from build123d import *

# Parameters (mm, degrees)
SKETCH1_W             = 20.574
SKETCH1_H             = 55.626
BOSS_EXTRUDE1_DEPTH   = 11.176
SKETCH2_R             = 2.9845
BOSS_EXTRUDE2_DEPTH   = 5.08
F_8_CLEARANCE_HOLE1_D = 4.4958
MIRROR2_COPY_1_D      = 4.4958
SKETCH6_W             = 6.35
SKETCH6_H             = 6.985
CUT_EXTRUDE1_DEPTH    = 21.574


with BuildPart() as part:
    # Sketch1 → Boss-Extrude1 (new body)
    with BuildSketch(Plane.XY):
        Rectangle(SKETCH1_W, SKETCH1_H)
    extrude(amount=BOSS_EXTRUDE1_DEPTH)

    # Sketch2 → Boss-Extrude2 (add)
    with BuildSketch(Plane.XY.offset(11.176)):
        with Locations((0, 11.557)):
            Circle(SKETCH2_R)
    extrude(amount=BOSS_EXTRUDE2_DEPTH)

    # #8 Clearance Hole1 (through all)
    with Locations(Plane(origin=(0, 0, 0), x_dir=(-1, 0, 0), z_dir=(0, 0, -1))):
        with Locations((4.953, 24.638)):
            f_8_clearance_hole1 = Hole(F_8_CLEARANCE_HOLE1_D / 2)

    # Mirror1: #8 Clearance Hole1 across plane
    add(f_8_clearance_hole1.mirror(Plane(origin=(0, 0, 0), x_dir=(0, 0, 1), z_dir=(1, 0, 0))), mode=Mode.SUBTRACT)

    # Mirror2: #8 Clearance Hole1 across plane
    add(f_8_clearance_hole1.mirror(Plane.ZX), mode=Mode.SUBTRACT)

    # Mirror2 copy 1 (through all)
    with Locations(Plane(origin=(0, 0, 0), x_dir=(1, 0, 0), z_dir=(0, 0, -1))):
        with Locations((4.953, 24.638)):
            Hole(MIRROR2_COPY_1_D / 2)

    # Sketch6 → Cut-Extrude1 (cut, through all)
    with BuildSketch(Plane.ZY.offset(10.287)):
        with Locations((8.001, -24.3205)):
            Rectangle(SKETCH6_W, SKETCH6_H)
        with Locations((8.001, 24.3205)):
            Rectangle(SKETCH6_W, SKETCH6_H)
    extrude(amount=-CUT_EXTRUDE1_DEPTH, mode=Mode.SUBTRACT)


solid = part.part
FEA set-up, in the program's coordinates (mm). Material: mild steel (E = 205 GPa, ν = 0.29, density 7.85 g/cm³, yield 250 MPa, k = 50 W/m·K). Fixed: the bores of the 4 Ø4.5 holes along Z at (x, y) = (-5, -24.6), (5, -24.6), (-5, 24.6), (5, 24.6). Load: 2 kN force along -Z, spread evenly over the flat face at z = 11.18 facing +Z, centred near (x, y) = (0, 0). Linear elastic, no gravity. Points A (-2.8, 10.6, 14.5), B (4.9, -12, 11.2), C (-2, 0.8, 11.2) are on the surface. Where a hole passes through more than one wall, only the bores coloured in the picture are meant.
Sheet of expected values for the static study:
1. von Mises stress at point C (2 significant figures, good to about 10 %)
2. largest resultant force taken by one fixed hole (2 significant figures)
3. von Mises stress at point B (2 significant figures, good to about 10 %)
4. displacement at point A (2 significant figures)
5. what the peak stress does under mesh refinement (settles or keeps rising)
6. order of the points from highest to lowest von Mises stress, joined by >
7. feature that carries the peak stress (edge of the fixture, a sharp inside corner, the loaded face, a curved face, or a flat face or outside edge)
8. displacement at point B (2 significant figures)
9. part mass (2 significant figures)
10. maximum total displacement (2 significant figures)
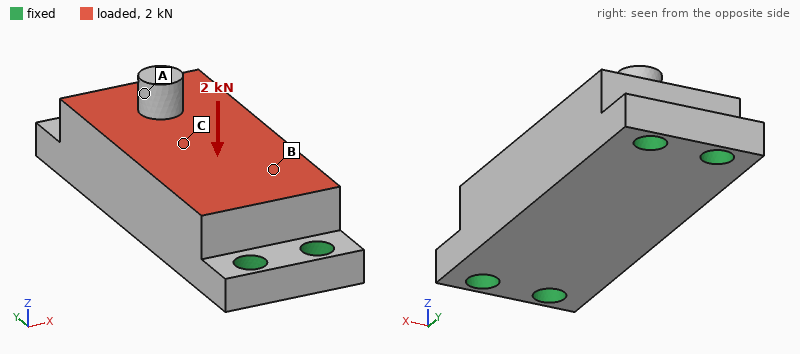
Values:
19 MPa
660 N
11 MPa
3.0 µm
keeps rising
C > B > A
edge of the fixture
2.7 µm
85 g
3.8 µm
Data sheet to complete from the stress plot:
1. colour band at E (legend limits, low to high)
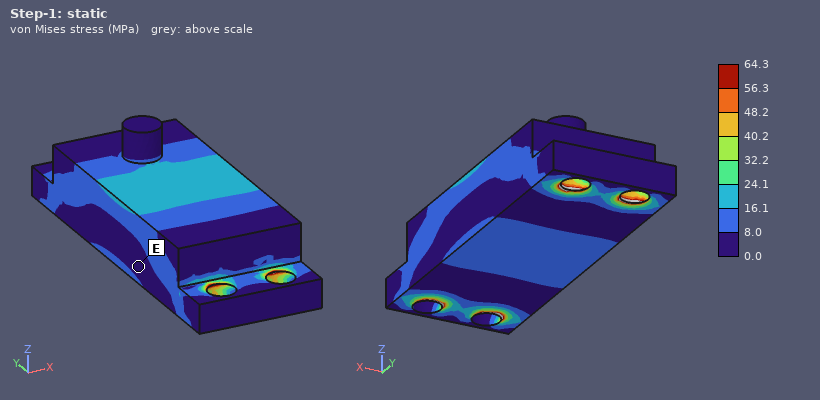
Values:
0.0 to 8.0 MPa
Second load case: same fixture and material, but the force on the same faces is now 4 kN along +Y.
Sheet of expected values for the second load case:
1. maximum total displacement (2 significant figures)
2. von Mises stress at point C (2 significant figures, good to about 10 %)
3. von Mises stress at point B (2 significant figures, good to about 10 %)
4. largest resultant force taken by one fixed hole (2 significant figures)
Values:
1.9 µm
8.4 MPa
8.8 MPa
1.1 kN
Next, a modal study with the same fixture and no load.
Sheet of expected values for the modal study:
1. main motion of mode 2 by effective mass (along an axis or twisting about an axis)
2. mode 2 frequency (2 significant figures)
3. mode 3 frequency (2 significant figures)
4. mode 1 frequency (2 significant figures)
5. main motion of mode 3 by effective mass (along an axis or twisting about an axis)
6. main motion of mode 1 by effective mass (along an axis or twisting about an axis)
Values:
along X
17 kHz
23 kHz
15 kHz
along X
along Z
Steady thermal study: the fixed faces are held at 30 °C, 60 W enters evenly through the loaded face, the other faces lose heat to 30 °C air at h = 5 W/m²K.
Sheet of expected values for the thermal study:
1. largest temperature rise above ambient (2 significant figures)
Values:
60 K
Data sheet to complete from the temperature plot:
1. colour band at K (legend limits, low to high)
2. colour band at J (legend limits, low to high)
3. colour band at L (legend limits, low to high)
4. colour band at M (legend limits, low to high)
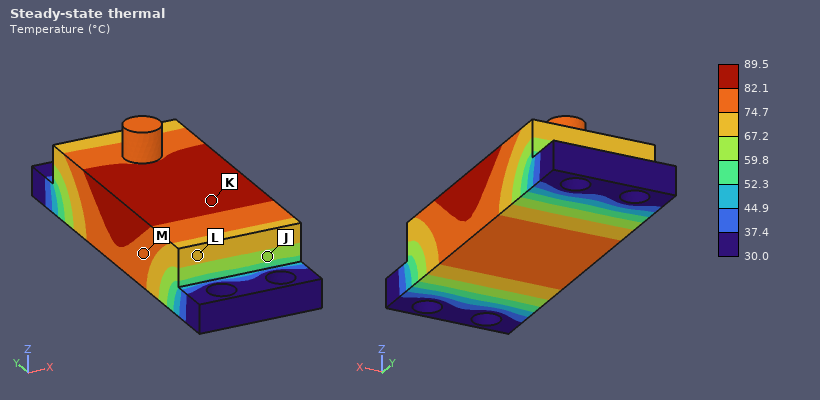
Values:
82.1 to 89.5 °C
59.8 to 67.2 °C
67.2 to 74.7 °C
74.7 to 82.1 °C
